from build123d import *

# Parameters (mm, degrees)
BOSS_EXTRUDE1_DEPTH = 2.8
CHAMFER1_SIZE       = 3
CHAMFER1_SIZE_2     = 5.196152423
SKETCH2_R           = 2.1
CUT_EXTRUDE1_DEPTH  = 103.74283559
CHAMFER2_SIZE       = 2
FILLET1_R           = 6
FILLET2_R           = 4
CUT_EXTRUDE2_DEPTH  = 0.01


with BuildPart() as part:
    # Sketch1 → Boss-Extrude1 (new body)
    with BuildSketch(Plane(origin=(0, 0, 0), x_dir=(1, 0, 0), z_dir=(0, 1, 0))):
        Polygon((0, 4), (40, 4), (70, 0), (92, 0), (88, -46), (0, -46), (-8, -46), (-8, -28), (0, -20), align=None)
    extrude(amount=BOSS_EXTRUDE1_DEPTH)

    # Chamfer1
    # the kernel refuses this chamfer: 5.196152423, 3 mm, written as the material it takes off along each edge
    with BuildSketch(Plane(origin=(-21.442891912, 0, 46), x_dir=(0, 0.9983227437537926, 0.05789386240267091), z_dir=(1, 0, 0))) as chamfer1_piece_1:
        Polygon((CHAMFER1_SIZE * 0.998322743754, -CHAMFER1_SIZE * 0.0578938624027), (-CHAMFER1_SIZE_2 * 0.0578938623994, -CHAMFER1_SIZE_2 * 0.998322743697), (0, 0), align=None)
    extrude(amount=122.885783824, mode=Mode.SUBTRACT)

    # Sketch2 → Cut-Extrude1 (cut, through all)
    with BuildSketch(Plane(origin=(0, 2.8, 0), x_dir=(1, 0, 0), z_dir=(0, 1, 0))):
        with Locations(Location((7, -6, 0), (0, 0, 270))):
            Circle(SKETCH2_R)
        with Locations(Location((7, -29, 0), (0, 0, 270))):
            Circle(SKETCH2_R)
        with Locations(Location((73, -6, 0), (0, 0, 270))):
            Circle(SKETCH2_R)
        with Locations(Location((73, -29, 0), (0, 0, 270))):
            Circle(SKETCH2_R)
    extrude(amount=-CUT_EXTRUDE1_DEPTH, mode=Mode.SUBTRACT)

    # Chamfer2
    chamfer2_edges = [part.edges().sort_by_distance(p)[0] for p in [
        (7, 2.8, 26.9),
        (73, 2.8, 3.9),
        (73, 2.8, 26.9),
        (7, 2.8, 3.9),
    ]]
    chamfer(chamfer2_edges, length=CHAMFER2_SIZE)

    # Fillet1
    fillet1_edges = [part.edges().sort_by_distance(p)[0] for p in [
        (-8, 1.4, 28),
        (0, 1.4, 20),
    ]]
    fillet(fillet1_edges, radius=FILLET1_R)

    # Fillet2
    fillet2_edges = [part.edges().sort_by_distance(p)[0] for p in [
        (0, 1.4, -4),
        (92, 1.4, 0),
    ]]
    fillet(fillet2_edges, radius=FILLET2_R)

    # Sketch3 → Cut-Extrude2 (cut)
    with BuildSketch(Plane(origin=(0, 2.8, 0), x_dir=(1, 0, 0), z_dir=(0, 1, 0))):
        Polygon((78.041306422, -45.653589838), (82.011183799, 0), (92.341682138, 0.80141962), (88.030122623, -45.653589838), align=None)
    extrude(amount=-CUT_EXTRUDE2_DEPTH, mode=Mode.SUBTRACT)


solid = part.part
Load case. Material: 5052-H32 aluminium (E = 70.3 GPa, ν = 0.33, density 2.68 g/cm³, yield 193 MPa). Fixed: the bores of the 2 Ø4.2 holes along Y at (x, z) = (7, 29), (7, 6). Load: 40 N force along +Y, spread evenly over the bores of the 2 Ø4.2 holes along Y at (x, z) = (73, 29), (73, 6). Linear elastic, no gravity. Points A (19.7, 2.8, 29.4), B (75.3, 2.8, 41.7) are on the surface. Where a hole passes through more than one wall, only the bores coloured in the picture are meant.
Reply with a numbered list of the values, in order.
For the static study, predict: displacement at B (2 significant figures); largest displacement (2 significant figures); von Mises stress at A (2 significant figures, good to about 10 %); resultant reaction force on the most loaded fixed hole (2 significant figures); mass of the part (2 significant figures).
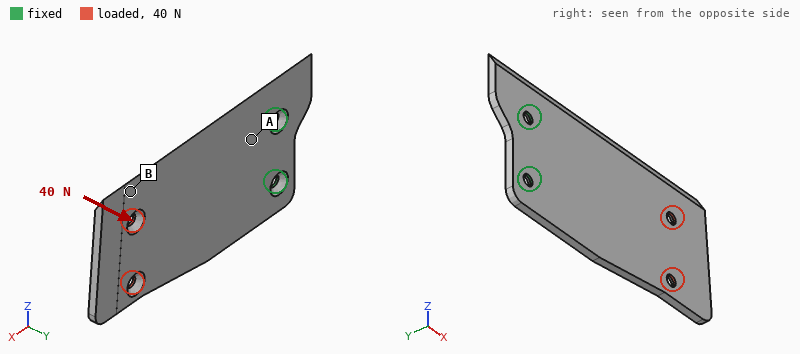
1. 0.86 mm
2. 1.2 mm
3. 28 MPa
4. 64 N
5. 31 g
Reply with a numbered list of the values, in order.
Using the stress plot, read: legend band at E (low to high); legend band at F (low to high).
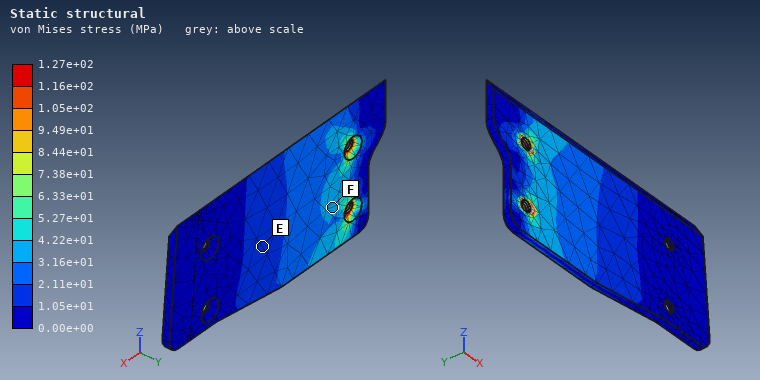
1. 1.05e+01 to 2.11e+01 MPa
2. 3.16e+01 to 4.22e+01 MPa
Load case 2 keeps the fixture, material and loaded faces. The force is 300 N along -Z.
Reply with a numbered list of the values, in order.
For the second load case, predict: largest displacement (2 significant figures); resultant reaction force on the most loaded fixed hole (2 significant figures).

1. 95 µm
2. 800 N
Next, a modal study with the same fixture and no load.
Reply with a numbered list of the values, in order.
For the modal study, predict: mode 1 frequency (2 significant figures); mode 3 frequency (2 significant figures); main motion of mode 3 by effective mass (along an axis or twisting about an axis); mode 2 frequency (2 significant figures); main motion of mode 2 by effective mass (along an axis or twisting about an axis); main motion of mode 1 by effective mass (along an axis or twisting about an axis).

1. 310 Hz
2. 1900 Hz
3. along Y
4. 1300 Hz
5. twisting about X
6. along Y
